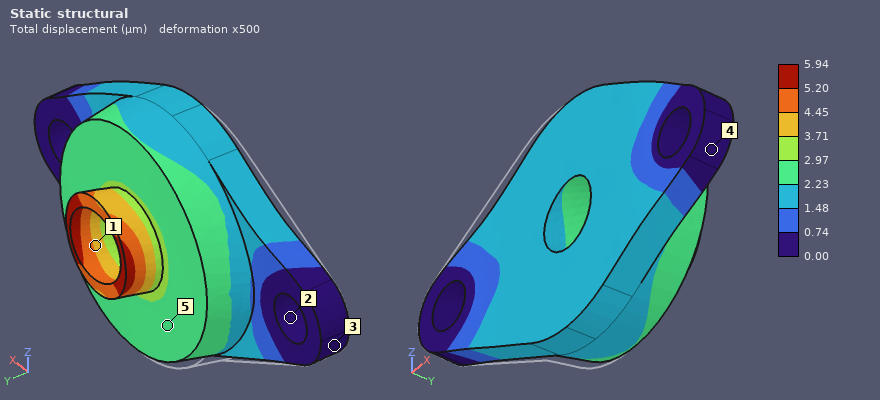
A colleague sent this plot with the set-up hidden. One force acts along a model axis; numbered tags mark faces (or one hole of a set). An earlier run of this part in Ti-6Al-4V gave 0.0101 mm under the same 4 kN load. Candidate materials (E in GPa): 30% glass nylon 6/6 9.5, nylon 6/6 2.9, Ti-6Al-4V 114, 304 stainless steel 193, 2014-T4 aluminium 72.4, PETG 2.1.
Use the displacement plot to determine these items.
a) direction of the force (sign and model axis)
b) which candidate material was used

+X
304 stainless steel
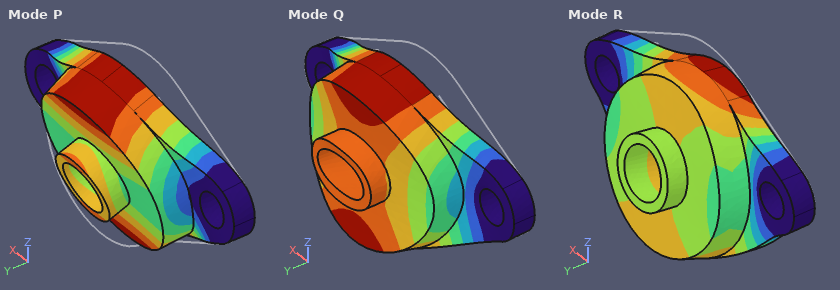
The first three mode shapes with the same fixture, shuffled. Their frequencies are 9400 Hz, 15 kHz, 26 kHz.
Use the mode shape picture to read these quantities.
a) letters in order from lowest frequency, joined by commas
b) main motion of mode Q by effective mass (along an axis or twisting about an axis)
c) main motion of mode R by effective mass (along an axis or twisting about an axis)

P, Q, R
along Y
along Z
